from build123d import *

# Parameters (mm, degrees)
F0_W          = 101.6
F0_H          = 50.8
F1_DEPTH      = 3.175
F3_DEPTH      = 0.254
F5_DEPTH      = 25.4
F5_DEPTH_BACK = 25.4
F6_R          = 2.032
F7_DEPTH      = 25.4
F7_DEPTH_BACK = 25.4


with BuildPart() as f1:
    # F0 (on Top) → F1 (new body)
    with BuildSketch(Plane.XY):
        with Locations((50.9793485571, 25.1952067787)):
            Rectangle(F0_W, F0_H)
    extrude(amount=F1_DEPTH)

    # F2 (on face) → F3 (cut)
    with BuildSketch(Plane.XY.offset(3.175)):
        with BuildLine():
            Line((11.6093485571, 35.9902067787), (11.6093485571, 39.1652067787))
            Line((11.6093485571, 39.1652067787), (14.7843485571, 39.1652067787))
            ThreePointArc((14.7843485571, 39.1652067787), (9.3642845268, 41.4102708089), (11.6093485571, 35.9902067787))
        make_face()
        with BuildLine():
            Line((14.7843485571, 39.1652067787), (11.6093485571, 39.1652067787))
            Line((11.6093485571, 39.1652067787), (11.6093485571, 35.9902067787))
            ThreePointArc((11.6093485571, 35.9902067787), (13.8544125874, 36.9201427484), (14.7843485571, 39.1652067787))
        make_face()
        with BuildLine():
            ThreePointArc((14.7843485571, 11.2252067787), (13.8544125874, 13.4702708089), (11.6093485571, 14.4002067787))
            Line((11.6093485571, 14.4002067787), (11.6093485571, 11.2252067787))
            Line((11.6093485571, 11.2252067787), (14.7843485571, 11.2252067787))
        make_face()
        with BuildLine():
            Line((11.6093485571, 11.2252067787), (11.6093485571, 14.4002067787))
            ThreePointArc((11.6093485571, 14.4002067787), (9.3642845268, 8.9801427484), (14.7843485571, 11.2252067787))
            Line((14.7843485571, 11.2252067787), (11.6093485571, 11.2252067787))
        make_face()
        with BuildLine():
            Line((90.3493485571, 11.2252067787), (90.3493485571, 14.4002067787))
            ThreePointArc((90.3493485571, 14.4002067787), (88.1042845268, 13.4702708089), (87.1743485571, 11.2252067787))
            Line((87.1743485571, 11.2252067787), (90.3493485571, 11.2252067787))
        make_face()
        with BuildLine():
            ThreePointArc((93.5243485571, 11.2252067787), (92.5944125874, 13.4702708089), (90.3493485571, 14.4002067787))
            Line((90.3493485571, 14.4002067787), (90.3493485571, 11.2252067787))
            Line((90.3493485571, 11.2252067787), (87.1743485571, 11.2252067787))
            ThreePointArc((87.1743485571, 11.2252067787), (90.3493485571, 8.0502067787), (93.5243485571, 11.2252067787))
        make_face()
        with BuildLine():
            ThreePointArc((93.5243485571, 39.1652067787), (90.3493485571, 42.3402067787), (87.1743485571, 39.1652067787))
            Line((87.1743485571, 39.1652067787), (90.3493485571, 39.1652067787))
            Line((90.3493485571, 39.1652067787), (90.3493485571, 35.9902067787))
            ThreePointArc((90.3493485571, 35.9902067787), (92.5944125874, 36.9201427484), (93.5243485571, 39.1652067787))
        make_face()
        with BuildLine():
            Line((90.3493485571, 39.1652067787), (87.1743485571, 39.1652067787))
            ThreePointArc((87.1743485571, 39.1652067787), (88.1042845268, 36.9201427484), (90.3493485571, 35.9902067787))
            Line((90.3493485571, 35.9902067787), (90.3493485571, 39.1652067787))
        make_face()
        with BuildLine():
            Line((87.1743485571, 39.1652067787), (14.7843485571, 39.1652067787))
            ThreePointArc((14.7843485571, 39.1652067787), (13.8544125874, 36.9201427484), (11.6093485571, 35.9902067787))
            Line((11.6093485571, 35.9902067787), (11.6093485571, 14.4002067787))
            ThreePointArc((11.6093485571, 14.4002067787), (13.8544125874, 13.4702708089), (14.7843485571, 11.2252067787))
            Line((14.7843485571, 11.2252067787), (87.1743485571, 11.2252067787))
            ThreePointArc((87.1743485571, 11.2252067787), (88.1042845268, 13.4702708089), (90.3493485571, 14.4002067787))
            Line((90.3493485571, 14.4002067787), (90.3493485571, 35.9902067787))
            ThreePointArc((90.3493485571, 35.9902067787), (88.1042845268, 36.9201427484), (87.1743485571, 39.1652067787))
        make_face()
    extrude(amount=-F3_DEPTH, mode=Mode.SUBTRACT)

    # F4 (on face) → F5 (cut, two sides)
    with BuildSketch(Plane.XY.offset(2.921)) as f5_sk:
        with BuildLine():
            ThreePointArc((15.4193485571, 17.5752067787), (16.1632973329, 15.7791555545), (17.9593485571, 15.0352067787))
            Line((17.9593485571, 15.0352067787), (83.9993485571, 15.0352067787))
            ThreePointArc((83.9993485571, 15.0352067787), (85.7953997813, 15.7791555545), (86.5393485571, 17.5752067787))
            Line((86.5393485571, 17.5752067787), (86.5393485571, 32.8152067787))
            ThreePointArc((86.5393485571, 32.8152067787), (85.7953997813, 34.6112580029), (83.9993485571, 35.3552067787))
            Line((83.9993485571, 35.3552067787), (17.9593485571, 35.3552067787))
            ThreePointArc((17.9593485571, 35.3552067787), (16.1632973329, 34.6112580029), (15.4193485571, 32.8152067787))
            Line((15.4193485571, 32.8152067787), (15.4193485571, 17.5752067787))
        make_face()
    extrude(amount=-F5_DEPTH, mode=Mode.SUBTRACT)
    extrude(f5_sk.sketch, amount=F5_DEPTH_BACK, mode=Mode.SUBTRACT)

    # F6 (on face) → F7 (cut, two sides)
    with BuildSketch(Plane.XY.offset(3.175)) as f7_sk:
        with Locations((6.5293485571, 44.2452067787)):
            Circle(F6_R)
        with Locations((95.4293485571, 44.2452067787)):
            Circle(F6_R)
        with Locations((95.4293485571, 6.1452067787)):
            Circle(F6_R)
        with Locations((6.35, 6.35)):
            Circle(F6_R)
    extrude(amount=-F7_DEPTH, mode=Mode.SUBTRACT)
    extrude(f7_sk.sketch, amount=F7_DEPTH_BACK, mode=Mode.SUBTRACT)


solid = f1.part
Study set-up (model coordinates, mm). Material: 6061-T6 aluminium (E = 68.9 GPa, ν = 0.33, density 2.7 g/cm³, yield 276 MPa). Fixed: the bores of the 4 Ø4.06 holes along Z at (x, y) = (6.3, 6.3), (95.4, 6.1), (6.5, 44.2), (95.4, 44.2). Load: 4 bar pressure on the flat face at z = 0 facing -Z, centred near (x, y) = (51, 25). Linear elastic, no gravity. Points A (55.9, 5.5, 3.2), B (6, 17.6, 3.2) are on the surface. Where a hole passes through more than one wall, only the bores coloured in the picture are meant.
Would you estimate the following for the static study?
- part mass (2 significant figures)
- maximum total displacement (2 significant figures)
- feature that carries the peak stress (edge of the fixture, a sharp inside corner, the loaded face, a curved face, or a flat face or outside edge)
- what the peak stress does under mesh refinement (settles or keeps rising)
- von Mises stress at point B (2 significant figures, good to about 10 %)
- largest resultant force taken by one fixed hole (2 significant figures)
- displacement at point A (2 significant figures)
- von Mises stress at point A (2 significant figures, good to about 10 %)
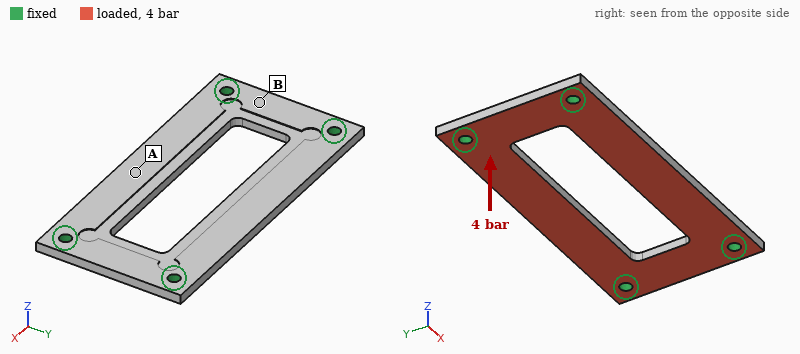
31 g
0.35 mm
edge of the fixture
keeps rising
27 MPa
370 N
0.33 mm
74 MPa
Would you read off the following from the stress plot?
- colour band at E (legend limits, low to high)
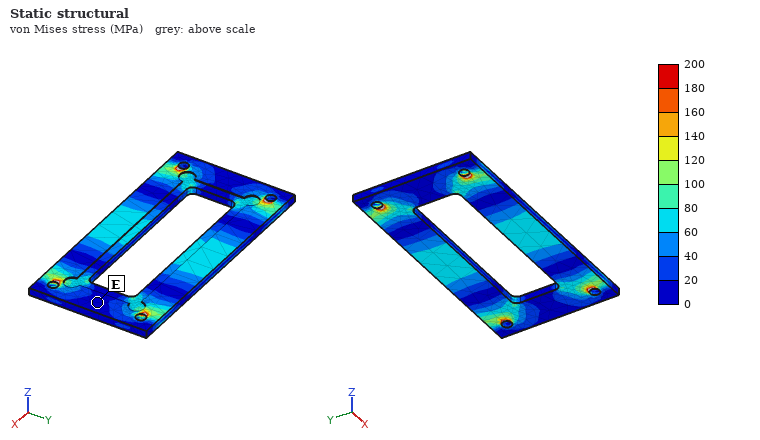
0 to 20 MPa
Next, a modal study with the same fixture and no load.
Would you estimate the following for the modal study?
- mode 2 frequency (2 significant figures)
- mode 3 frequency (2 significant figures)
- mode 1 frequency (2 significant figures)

2200 Hz
5800 Hz
2200 Hz
